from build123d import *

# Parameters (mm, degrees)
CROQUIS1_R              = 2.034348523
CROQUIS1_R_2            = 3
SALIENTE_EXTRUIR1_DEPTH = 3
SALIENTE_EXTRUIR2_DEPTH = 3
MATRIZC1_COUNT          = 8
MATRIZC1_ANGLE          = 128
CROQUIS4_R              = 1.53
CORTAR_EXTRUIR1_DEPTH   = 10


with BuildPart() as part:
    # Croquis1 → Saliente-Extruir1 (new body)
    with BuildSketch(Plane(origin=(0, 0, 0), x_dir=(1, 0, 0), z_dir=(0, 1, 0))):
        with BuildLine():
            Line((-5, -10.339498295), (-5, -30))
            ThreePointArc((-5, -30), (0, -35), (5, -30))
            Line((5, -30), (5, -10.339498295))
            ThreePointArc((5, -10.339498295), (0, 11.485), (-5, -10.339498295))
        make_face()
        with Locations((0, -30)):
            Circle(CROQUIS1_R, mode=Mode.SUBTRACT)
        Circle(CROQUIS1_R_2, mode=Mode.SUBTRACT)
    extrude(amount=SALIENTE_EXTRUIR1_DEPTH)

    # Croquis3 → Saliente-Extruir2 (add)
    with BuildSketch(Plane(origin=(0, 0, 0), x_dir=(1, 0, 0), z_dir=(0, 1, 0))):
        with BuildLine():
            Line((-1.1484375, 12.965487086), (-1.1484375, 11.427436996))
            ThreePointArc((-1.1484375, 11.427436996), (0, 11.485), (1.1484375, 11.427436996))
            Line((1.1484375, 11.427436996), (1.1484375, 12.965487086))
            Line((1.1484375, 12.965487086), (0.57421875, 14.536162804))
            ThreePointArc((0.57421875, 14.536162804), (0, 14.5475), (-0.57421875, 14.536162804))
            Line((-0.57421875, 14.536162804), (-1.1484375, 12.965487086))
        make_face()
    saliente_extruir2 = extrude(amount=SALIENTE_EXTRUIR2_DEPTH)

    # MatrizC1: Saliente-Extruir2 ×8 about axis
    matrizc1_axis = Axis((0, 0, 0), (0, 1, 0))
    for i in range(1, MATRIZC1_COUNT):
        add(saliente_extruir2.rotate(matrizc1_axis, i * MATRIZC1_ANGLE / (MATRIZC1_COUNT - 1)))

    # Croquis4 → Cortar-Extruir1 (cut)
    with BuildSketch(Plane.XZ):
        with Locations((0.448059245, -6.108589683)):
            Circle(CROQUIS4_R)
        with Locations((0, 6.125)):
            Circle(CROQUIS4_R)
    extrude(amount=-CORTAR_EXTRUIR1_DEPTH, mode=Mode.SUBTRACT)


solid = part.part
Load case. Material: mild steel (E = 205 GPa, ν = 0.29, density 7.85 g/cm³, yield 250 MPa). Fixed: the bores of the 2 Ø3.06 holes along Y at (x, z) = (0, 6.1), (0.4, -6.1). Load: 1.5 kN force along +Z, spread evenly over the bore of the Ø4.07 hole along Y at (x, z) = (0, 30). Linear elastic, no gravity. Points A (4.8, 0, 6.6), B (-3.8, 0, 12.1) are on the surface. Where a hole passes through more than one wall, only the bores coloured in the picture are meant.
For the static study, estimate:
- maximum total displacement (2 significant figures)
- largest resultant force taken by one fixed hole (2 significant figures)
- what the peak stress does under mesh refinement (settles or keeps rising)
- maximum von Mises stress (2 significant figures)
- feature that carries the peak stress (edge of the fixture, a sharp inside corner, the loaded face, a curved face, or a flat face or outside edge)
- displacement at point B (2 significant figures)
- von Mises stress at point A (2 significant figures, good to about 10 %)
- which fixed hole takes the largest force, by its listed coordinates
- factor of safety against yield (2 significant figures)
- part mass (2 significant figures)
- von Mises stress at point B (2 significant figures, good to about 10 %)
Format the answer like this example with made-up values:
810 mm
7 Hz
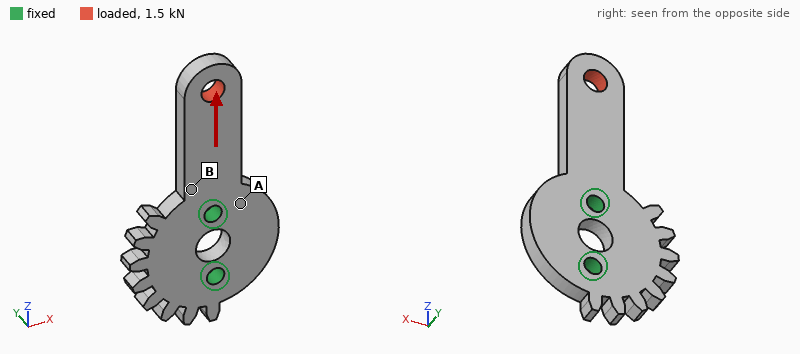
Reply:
7.7 µm
1.3 kN
settles
140 MPa
the loaded face
1.5 µm
18 MPa
(0, 6.1)
1.8
15 g
47 MPa
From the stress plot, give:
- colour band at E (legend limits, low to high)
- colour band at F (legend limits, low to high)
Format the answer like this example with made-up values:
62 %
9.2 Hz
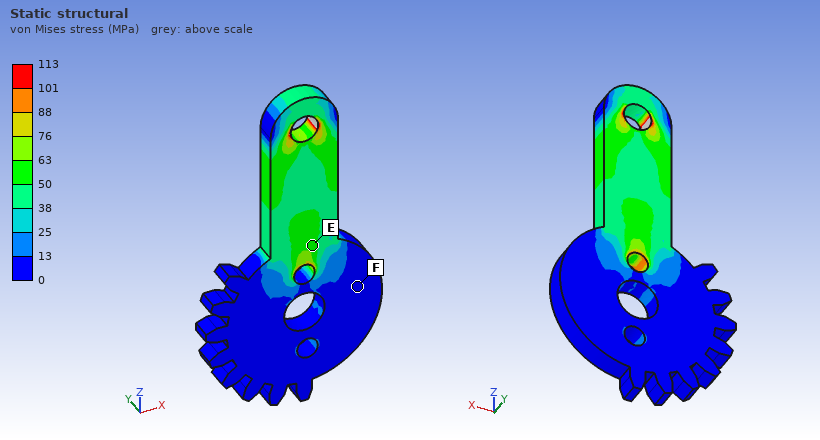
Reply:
50 to 63 MPa
0 to 13 MPa
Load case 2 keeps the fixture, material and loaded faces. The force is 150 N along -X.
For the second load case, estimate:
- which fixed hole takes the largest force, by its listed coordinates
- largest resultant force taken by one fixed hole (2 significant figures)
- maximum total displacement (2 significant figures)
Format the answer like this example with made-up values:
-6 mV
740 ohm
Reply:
(0, 6.1)
310 N
20 µm
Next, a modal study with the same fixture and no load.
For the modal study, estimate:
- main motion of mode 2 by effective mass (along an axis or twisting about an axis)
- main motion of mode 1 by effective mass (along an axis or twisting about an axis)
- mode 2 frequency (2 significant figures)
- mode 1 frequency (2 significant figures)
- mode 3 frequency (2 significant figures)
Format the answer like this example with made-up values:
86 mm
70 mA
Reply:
along X
along Y
10 kHz
3600 Hz
16 kHz
